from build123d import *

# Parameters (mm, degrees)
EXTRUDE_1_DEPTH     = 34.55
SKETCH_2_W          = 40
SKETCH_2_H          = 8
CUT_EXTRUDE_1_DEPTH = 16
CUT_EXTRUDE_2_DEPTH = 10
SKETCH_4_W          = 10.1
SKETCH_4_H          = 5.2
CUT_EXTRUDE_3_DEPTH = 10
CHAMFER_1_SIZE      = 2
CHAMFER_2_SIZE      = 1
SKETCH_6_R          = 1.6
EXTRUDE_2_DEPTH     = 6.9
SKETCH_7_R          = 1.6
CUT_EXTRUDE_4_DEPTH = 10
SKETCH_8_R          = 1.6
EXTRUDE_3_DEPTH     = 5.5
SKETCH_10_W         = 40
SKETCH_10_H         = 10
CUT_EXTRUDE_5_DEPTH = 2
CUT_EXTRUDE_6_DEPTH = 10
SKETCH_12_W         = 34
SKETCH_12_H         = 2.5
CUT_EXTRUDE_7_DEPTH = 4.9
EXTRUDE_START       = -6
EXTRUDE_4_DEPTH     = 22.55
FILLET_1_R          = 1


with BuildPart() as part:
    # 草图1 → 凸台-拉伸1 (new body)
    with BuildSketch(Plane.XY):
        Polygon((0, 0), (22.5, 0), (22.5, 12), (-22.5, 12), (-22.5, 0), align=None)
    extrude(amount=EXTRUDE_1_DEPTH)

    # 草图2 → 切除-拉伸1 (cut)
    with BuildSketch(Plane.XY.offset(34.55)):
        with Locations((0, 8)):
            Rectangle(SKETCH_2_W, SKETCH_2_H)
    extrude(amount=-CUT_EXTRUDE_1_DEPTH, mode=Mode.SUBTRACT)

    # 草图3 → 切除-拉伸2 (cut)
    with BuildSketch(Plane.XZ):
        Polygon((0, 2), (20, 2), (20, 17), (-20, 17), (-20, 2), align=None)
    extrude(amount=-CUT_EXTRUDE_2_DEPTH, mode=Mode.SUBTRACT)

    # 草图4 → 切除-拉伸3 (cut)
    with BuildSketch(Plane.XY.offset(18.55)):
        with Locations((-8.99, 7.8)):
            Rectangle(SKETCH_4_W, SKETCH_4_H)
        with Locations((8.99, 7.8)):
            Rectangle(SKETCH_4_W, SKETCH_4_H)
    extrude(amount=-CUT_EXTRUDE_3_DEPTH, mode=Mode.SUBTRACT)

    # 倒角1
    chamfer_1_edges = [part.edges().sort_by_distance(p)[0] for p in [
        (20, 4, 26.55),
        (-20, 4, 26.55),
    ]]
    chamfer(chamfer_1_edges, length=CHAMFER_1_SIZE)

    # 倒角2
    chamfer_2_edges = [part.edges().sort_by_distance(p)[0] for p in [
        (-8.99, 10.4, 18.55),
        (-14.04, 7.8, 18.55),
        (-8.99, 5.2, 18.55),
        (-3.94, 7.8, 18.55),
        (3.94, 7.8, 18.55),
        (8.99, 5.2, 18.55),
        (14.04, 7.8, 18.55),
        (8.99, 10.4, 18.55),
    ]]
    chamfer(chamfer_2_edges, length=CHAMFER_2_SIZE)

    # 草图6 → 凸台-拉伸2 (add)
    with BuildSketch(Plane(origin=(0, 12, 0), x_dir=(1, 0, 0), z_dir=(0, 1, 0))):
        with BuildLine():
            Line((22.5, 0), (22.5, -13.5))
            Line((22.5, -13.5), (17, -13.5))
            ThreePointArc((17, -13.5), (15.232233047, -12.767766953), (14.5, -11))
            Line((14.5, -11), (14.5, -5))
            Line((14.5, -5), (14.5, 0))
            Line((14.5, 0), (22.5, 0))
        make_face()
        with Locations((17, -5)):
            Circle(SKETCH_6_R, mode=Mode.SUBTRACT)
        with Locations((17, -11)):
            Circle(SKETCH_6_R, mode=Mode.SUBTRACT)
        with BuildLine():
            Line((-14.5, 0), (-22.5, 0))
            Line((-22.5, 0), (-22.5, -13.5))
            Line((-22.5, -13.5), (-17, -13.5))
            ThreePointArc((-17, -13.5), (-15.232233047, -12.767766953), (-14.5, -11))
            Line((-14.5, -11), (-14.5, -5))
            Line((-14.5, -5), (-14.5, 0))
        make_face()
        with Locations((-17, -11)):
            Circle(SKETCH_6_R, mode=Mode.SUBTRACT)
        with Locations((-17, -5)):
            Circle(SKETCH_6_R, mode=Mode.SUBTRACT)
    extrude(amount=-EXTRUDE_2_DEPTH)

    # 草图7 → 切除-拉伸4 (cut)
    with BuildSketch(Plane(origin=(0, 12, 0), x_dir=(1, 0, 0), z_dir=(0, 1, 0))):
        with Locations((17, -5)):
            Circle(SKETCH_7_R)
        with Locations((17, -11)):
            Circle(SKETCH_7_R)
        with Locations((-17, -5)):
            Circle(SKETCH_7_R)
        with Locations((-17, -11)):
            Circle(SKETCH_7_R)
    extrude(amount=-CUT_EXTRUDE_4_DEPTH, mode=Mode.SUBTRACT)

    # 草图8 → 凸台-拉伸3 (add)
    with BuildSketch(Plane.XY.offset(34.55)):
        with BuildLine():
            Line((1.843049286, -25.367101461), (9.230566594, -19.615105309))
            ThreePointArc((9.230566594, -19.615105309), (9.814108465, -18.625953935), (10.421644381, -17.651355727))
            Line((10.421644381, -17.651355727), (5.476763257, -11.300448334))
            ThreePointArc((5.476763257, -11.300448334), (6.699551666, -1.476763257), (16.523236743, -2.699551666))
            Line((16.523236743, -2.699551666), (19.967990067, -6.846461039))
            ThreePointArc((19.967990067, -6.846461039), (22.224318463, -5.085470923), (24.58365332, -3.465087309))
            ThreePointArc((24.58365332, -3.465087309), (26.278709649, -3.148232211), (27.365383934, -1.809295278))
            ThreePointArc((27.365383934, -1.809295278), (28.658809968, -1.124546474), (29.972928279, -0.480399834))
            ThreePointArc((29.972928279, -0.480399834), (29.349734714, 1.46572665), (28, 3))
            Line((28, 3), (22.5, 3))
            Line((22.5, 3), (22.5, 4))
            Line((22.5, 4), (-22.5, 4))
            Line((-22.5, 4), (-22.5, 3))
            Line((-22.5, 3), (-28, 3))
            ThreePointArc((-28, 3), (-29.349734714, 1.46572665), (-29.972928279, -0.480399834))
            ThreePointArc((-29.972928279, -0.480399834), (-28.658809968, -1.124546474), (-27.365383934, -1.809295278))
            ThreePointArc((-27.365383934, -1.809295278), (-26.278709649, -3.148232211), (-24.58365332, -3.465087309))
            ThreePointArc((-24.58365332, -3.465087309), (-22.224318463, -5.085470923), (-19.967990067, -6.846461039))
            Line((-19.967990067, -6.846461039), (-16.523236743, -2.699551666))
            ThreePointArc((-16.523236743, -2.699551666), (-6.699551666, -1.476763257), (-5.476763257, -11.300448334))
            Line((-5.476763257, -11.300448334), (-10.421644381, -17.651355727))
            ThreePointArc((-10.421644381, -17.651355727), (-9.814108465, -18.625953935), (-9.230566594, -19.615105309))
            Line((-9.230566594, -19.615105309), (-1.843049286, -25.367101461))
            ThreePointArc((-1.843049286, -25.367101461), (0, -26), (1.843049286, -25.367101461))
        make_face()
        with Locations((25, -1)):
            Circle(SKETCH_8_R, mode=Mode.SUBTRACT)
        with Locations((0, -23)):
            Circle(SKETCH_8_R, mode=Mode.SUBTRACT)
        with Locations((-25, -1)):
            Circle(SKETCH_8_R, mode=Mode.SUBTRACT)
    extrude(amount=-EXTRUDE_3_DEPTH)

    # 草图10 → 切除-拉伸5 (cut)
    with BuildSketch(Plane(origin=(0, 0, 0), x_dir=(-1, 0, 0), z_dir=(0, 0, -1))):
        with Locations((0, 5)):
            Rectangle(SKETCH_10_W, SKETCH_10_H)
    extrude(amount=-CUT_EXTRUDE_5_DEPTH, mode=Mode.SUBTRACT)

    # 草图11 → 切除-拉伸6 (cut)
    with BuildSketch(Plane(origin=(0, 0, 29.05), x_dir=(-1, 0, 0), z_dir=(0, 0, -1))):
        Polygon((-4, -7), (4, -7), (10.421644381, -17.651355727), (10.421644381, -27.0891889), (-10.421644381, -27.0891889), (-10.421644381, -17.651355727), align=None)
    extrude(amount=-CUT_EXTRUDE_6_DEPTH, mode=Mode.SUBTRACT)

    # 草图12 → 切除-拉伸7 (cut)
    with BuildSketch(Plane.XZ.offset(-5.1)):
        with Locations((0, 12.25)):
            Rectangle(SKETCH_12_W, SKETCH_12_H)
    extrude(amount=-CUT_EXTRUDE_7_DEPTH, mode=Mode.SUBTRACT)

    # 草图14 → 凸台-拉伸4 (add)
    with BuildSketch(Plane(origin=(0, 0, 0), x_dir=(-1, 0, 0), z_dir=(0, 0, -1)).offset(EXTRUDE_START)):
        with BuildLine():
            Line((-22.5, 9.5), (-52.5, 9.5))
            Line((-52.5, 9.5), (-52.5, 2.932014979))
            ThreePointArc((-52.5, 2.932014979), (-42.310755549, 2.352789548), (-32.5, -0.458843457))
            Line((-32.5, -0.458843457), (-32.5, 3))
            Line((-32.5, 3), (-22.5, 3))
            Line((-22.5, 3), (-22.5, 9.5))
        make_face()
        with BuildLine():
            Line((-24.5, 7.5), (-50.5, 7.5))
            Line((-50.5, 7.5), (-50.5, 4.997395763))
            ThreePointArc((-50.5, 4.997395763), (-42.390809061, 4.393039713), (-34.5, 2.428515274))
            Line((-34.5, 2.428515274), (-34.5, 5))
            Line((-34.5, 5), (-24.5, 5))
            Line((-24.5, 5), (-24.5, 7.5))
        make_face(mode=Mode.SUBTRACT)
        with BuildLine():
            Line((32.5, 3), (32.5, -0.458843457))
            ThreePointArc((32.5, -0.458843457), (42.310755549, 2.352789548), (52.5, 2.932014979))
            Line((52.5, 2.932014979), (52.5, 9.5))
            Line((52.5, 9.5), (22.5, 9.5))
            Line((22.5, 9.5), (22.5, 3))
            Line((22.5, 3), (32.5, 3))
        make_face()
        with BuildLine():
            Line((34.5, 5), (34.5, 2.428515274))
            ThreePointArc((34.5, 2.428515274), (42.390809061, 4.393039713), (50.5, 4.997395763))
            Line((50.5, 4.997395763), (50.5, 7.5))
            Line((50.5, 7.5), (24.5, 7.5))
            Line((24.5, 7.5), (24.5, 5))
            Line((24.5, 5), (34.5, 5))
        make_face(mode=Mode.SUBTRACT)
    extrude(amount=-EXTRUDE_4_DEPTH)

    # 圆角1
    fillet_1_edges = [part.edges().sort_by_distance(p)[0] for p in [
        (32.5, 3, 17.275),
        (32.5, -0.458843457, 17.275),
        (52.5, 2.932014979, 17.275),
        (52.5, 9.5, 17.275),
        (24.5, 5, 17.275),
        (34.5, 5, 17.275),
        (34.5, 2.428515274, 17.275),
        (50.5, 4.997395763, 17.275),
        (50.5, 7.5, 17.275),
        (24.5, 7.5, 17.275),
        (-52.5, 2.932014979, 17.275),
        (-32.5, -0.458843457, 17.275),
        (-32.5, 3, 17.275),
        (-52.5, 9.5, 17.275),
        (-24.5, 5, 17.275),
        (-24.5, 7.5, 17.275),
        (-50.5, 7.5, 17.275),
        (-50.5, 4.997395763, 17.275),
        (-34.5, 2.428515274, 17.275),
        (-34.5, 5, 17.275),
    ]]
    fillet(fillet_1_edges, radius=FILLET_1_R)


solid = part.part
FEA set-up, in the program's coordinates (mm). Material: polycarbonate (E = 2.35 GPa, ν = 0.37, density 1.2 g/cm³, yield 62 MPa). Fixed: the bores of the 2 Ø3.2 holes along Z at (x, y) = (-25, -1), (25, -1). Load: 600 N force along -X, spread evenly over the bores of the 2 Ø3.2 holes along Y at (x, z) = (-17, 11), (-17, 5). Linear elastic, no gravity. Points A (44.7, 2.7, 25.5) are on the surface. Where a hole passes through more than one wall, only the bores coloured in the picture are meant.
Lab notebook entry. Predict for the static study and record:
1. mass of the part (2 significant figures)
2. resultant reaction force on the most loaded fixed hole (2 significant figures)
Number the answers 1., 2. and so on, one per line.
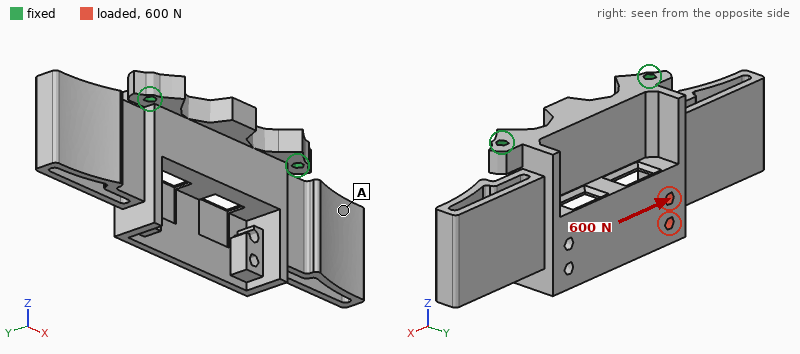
1. 17 g
2. 460 N
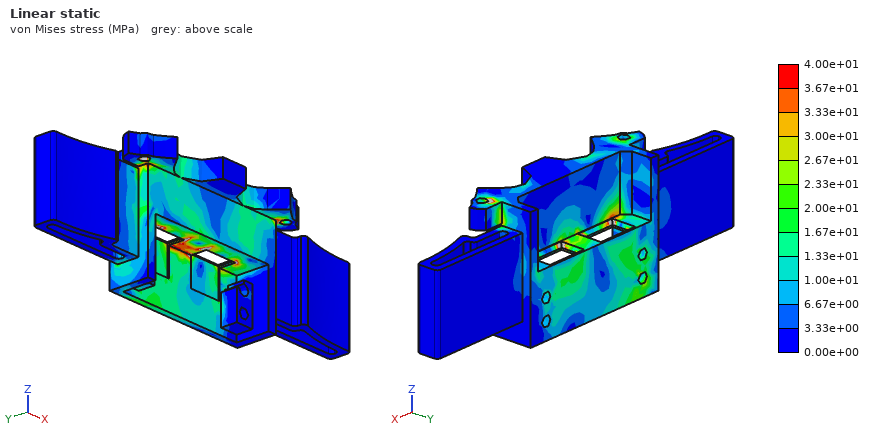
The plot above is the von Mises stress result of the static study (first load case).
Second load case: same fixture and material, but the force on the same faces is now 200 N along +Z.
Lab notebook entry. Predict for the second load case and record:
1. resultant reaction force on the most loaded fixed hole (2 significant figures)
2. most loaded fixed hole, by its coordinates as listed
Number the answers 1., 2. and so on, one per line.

1. 180 N
2. (-25, -1)
